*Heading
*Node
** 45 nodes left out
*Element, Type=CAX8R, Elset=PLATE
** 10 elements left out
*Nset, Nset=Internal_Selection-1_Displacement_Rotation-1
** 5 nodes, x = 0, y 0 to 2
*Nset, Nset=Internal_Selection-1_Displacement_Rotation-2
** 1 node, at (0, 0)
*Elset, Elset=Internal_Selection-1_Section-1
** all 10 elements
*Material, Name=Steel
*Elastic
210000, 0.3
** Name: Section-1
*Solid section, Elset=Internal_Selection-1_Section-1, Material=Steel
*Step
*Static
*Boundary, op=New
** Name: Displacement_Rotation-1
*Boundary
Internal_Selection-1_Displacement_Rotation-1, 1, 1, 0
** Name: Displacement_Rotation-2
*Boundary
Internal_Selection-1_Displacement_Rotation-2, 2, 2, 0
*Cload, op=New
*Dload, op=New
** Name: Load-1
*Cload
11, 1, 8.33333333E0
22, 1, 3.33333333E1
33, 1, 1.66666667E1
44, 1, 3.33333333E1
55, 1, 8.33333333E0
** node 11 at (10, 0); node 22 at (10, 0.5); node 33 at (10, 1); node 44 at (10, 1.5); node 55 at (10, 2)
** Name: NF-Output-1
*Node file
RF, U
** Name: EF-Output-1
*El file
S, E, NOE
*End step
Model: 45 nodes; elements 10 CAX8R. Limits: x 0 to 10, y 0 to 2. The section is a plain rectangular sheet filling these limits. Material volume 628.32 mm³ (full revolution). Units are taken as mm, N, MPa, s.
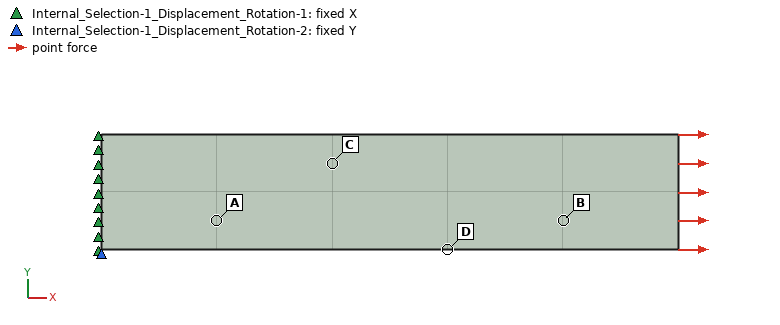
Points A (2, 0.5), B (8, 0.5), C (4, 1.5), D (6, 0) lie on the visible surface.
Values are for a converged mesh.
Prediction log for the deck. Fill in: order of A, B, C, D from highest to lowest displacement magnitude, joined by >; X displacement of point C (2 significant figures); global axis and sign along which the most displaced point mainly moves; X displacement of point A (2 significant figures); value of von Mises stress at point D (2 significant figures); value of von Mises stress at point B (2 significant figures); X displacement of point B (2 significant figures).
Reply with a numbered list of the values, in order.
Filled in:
1. B > D > C > A
2. 1.1e-05 mm
3. +X
4. 5.3e-06 mm
5. 0.80 MPa
6. 0.81 MPa
7. 2.1e-05 mm
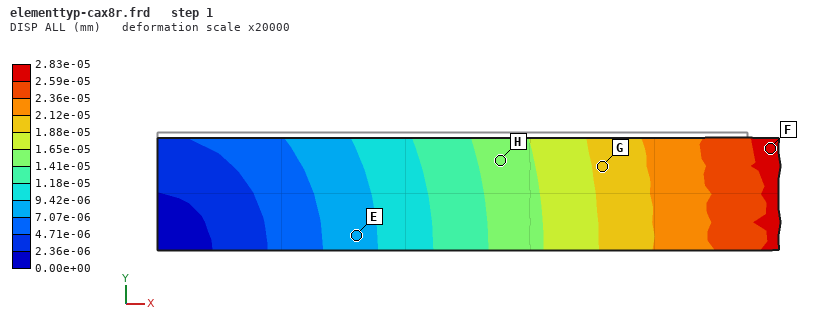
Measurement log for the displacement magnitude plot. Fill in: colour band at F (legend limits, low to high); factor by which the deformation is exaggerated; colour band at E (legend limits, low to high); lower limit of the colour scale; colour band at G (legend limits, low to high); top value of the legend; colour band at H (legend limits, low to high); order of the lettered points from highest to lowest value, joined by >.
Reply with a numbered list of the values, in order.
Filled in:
1. 2.59e-05 to 2.83e-05 mm
2. 20000
3. 7.07e-06 to 9.42e-06 mm
4. 0.00e+00 mm
5. 1.88e-05 to 2.12e-05 mm
6. 2.83e-05 mm
7. 1.41e-05 to 1.65e-05 mm
8. F > G > H > E
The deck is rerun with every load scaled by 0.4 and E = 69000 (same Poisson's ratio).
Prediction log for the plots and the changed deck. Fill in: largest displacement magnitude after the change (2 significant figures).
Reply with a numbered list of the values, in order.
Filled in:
1. 3.4e-05 mm
